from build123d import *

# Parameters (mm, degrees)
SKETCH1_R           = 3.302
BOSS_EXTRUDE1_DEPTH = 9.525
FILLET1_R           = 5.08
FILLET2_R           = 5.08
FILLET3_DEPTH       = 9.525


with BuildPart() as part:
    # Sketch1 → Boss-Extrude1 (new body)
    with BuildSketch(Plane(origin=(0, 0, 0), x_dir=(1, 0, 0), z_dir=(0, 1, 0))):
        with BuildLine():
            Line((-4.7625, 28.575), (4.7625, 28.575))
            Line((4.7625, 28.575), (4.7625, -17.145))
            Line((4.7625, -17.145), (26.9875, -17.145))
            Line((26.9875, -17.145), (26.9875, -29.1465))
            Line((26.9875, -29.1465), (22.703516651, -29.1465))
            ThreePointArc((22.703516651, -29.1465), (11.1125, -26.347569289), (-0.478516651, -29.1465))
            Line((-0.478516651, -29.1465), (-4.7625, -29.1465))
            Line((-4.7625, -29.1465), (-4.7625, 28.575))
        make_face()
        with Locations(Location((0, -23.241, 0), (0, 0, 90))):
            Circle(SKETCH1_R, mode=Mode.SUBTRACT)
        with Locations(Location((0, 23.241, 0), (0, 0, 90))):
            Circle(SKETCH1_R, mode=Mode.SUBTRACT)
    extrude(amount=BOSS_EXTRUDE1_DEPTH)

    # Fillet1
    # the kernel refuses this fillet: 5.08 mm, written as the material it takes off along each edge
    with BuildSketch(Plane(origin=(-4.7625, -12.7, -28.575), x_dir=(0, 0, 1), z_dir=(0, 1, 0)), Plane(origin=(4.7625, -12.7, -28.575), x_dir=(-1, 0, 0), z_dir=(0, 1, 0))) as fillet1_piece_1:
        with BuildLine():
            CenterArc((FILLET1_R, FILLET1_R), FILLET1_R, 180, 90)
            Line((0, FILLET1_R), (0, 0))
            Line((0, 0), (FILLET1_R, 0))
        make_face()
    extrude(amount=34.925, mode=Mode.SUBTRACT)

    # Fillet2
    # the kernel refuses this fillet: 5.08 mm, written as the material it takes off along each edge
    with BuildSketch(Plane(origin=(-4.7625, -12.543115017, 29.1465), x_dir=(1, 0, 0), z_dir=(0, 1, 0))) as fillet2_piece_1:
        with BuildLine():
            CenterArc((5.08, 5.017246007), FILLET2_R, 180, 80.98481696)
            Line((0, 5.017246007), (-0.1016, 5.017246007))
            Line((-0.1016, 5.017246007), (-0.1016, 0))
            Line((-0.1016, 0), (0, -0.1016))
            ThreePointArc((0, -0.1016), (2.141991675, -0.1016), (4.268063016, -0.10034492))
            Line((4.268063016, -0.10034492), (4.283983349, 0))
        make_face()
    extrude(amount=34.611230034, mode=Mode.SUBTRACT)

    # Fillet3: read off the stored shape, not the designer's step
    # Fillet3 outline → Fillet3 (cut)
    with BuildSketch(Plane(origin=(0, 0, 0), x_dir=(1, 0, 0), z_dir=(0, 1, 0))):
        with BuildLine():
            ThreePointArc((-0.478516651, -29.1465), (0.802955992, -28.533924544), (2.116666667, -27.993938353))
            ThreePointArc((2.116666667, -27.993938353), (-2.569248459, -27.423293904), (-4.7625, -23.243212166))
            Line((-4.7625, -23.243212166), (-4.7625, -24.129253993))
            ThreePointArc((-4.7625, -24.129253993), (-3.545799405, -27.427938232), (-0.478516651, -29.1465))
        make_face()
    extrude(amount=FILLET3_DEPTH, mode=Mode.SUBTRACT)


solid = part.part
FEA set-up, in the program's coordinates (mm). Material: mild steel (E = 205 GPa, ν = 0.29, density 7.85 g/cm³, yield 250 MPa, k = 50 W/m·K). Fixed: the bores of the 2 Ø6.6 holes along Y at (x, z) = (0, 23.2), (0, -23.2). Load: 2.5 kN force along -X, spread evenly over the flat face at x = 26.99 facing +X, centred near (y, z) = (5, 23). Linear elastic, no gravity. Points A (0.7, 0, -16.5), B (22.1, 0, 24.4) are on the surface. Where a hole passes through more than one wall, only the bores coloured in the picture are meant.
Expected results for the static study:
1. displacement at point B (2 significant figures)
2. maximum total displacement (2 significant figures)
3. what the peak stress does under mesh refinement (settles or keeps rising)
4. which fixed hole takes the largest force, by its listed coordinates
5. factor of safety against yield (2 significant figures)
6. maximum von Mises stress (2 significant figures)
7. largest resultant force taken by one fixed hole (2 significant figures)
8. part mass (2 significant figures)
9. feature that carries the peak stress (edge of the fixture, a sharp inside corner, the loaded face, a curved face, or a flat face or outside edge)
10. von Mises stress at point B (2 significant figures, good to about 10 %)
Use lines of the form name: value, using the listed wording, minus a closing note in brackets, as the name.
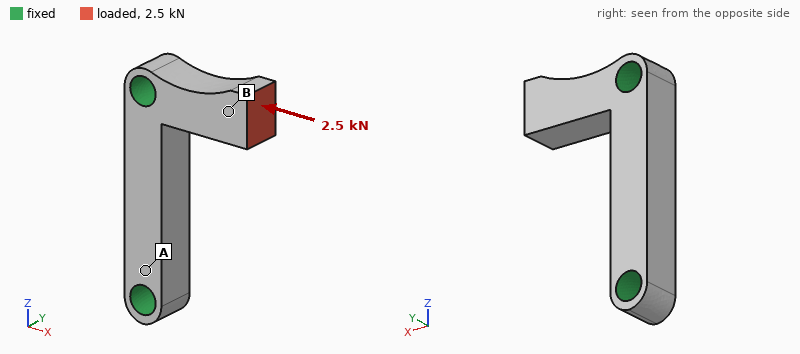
displacement at point B: 5.1 µm
maximum total displacement: 8.2 µm
what the peak stress does under mesh refinement: settles
which fixed hole takes the largest force, by its listed coordinates: (0, 23.2)
factor of safety against yield: 4.2
maximum von Mises stress: 60 MPa
largest resultant force taken by one fixed hole: 2.5 kN
part mass: 51 g
feature that carries the peak stress: a curved face
von Mises stress at point B: 27 MPa
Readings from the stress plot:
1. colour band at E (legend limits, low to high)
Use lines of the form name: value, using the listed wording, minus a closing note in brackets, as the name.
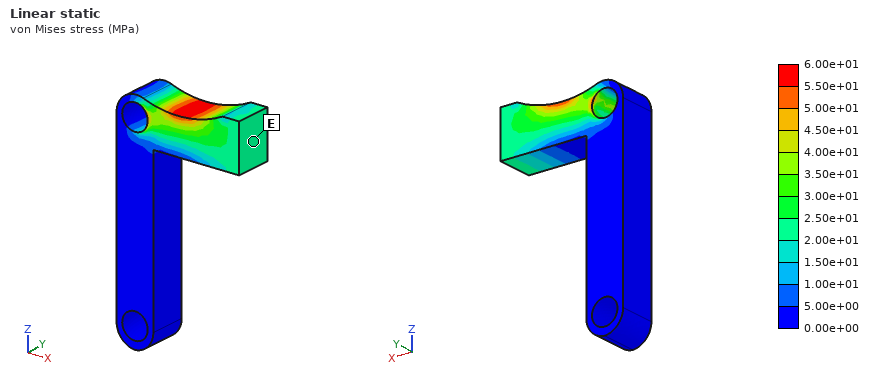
colour band at E: 2.00e+01 to 2.50e+01 MPa
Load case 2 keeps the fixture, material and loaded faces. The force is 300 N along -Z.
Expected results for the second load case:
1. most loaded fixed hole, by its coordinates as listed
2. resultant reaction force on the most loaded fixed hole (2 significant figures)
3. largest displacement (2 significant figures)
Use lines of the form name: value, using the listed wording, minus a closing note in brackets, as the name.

most loaded fixed hole, by its coordinates as listed: (0, 23.2)
resultant reaction force on the most loaded fixed hole: 260 N
largest displacement: 13 µm
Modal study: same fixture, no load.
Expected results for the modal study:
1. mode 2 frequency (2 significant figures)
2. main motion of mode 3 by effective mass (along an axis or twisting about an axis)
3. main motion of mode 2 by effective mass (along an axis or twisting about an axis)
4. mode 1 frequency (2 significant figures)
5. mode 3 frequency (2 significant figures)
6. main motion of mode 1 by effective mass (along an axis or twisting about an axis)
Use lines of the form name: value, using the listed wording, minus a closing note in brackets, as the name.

mode 2 frequency: 11 kHz
main motion of mode 3 by effective mass: along X
main motion of mode 2 by effective mass: along Y
mode 1 frequency: 10 kHz
mode 3 frequency: 22 kHz
main motion of mode 1 by effective mass: along Z
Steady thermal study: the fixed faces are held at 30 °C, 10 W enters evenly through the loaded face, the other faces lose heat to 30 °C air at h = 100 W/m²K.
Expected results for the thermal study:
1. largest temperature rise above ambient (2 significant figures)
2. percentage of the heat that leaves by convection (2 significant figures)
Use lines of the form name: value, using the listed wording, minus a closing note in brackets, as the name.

largest temperature rise above ambient: 43 K
percentage of the heat that leaves by convection: 22 %
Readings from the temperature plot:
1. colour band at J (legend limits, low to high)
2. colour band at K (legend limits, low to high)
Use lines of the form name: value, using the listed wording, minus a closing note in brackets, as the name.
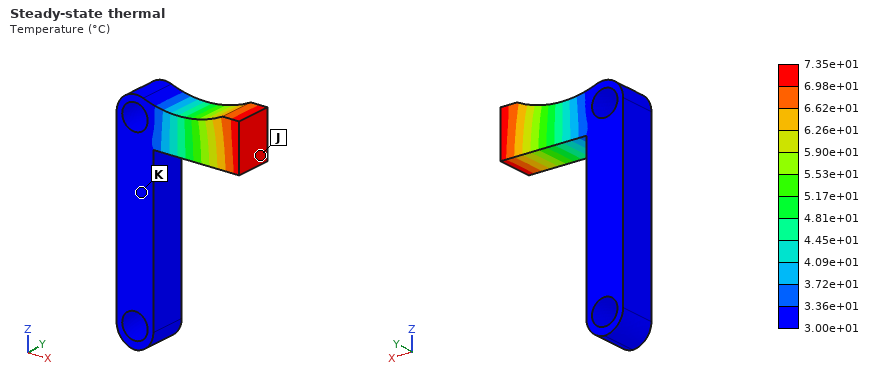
colour band at J: 6.98e+01 to 7.35e+01 °C
colour band at K: 3.00e+01 to 3.36e+01 °C
